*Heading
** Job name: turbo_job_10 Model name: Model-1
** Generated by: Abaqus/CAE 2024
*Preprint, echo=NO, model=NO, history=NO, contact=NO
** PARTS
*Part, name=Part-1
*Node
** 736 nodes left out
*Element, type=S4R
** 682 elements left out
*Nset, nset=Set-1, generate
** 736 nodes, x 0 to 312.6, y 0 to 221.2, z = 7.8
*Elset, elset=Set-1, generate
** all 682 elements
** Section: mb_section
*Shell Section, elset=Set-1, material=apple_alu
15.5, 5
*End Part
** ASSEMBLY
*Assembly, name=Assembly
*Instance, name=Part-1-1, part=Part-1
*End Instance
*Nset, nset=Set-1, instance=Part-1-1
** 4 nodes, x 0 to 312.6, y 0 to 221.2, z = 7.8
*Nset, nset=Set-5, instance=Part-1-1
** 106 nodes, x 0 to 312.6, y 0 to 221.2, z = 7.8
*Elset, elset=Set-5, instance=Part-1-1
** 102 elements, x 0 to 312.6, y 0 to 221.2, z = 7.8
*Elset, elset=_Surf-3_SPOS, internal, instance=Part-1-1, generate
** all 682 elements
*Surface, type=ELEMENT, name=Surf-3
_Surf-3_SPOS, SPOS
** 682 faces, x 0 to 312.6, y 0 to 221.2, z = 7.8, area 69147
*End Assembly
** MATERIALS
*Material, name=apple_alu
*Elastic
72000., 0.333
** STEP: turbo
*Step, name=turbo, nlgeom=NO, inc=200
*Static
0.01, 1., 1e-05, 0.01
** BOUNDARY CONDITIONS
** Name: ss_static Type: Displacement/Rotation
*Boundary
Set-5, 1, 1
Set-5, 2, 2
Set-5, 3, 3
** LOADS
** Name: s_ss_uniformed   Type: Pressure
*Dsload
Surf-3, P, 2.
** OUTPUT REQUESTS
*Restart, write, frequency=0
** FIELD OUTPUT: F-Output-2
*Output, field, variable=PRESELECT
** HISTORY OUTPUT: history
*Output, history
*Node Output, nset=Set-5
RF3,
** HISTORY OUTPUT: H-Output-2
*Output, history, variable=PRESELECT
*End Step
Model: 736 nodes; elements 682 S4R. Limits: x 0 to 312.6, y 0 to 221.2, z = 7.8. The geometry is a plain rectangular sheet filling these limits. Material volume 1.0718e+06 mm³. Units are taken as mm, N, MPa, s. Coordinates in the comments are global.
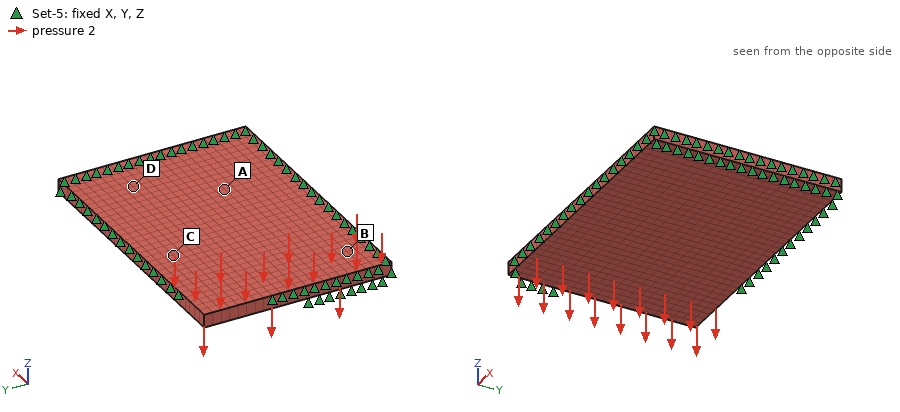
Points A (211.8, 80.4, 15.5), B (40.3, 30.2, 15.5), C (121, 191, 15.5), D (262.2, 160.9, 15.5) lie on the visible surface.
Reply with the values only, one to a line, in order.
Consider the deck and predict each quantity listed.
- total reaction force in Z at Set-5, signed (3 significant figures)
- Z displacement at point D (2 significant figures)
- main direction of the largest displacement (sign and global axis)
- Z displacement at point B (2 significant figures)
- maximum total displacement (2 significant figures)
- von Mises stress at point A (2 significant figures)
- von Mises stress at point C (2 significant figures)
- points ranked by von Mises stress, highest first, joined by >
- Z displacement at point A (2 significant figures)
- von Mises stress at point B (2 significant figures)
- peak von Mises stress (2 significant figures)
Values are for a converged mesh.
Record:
1.38e+05 N
-0.58 mm
-Z
-0.27 mm
1.4 mm
150 MPa
95 MPa
A > B > D > C
-1.1 mm
140 MPa
170 MPa
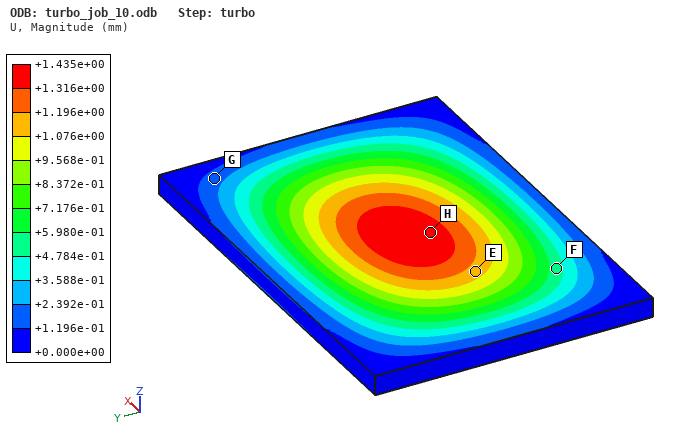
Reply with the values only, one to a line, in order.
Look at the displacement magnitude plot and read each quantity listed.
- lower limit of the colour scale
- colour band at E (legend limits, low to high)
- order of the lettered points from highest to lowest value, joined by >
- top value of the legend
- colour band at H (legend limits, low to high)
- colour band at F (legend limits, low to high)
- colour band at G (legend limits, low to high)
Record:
+0.000e+00 mm
+1.076e+00 to +1.196e+00 mm
H > E > F > G
+1.435e+00 mm
+1.316e+00 to +1.435e+00 mm
+4.784e-01 to +5.980e-01 mm
+1.196e-01 to +2.392e-01 mm
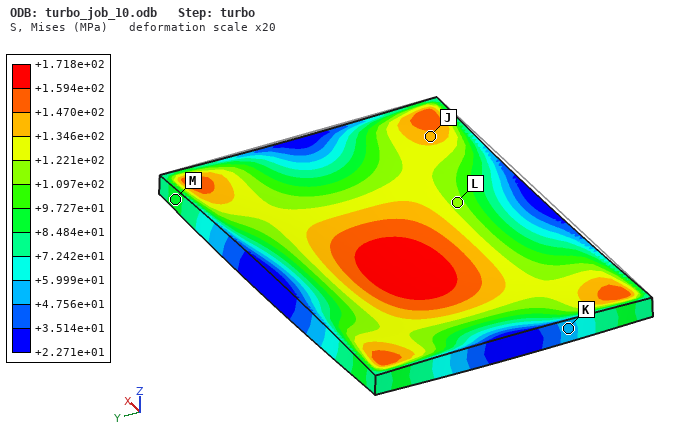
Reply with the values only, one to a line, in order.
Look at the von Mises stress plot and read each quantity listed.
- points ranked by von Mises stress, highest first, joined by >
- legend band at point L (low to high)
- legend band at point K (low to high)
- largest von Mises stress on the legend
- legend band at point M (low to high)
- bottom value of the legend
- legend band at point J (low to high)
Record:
J > L > M > K
+1.097e+02 to +1.221e+02 MPa
+4.756e+01 to +5.999e+01 MPa
+1.718e+02 MPa
+8.484e+01 to +9.727e+01 MPa
+2.271e+01 MPa
+1.346e+02 to +1.470e+02 MPa
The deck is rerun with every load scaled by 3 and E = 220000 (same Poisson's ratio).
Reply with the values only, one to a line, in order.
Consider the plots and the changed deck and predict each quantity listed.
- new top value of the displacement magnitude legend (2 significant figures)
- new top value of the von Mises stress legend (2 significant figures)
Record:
1.4 mm
520 MPa
